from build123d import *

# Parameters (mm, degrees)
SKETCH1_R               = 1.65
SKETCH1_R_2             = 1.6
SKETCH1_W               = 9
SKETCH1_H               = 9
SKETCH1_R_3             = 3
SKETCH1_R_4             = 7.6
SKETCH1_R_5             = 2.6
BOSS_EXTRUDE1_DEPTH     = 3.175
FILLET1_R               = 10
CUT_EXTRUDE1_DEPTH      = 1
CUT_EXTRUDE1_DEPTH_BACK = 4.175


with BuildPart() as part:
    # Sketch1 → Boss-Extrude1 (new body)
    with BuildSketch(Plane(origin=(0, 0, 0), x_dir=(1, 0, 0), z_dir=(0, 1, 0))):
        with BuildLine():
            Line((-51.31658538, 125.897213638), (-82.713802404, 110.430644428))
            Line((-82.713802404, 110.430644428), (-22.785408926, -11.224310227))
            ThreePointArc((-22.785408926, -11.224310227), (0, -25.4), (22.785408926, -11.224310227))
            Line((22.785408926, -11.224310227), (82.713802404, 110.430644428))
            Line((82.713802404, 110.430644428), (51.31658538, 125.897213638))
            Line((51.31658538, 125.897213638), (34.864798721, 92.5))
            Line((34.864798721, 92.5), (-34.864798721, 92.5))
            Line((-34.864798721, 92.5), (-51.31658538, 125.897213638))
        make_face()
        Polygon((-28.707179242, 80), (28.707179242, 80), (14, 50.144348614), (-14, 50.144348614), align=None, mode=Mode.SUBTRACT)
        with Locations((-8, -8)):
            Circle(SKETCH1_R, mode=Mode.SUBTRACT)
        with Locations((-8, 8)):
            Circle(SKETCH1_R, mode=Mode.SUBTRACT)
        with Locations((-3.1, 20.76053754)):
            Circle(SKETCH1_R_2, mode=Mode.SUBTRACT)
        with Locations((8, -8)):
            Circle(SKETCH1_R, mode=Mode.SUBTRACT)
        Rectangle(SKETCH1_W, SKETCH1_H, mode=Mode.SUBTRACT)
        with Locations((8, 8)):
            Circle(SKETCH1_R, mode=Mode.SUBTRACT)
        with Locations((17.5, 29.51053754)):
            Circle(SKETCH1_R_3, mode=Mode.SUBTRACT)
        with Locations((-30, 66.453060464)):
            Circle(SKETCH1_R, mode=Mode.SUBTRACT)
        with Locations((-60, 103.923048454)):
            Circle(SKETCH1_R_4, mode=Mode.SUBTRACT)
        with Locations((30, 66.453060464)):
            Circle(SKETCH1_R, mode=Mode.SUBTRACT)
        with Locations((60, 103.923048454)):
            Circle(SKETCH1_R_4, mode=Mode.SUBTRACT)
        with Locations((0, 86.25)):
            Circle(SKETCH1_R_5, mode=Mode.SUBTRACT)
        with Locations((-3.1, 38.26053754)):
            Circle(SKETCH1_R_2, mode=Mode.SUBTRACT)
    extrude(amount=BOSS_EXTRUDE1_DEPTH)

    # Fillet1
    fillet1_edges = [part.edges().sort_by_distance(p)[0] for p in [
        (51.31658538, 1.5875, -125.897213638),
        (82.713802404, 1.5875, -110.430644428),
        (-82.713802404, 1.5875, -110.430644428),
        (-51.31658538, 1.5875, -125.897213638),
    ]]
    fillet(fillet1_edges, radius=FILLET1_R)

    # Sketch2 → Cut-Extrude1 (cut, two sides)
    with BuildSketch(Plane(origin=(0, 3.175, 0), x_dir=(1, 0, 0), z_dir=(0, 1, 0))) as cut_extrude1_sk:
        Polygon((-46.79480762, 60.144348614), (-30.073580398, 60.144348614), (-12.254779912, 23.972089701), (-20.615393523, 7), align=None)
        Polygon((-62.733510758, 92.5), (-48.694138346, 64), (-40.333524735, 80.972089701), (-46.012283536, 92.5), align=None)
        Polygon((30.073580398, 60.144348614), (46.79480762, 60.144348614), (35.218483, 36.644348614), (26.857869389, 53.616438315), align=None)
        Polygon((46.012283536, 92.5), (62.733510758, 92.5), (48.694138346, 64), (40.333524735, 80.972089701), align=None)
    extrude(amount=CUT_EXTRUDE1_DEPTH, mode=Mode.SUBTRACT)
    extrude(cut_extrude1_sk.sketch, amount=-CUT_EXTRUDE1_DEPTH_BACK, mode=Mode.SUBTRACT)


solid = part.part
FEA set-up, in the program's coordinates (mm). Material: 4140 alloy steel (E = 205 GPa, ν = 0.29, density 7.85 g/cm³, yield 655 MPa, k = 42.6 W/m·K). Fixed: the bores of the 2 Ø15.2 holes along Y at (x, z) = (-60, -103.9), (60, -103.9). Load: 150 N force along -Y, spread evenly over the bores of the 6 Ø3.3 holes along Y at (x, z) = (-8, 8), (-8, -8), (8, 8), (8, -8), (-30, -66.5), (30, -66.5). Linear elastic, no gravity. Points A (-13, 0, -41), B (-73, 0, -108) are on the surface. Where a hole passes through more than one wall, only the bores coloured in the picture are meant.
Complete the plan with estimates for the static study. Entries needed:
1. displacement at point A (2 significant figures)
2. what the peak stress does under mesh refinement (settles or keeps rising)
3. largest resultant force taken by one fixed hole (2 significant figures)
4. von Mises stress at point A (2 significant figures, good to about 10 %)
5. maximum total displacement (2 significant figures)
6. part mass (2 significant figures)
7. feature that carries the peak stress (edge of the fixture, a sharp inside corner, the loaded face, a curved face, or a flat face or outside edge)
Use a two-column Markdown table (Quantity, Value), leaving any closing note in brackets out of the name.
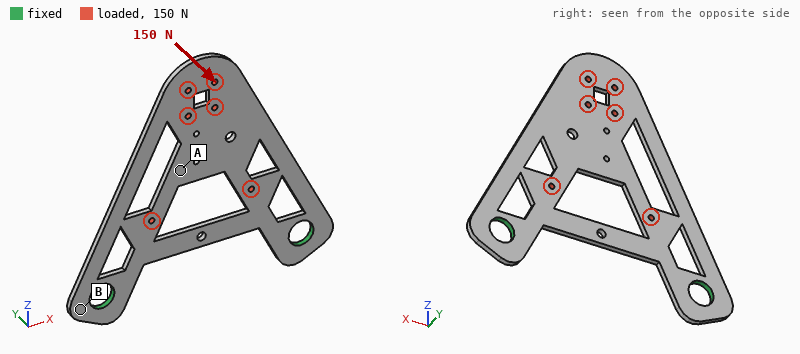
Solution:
| Quantity | Value |
|---|---|
| displacement at point A | 0.74 mm |
| what the peak stress does under mesh refinement | keeps rising |
| largest resultant force taken by one fixed hole | 76 N |
| von Mises stress at point A | 42 MPa |
| maximum total displacement | 2.1 mm |
| part mass | 220 g |
| feature that carries the peak stress | a sharp inside corner |
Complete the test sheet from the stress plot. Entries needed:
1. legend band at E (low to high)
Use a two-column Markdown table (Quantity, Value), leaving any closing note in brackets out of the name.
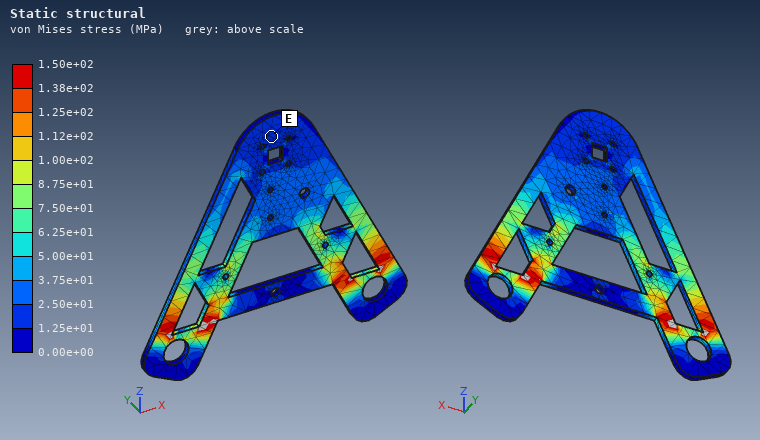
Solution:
| Quantity | Value |
|---|---|
| legend band at E | 1.25e+01 to 2.50e+01 MPa |
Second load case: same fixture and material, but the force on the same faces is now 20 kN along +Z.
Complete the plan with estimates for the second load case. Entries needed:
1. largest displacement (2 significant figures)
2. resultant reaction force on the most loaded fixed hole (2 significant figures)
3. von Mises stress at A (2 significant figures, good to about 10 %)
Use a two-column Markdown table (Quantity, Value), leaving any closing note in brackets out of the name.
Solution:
| Quantity | Value |
|---|---|
| largest displacement | 87 µm |
| resultant reaction force on the most loaded fixed hole | 11 kN |
| von Mises stress at A | 87 MPa |
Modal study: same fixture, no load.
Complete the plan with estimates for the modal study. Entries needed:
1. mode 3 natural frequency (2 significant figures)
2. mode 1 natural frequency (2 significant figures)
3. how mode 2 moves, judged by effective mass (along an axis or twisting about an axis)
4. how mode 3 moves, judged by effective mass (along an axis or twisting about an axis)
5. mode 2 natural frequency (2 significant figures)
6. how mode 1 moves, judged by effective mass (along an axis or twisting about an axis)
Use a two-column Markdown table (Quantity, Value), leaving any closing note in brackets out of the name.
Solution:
| Quantity | Value |
|---|---|
| mode 3 natural frequency | 870 Hz |
| mode 1 natural frequency | 160 Hz |
| how mode 2 moves, judged by effective mass | twisting about Z |
| how mode 3 moves, judged by effective mass | along Y |
| mode 2 natural frequency | 750 Hz |
| how mode 1 moves, judged by effective mass | along Y |
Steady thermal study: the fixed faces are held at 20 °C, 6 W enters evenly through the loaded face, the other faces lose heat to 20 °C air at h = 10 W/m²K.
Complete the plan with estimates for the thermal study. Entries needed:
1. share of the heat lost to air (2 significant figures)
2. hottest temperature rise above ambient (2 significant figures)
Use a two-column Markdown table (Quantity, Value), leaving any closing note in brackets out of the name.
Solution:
| Quantity | Value |
|---|---|
| share of the heat lost to air | 63 % |
| hottest temperature rise above ambient | 38 K |
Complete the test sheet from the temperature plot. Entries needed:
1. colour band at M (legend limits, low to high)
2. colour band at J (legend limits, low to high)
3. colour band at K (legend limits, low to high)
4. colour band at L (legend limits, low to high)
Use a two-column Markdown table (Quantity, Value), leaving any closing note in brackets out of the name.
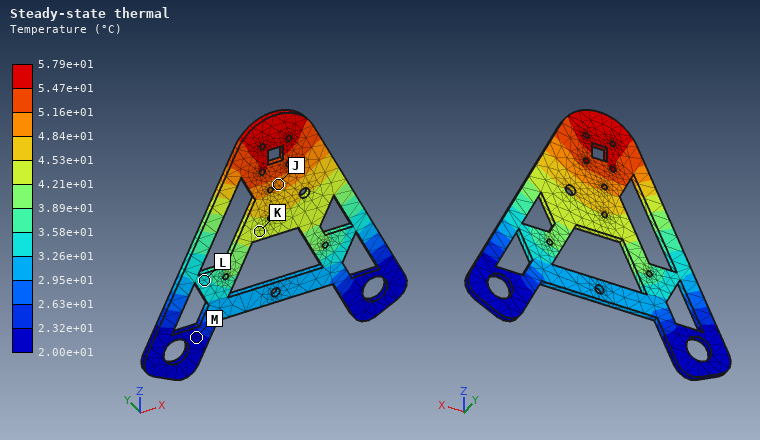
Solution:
| Quantity | Value |
|---|---|
| colour band at M | 2.00e+01 to 2.32e+01 °C |
| colour band at J | 4.84e+01 to 5.16e+01 °C |
| colour band at K | 4.21e+01 to 4.53e+01 °C |
| colour band at L | 3.26e+01 to 3.58e+01 °C |
